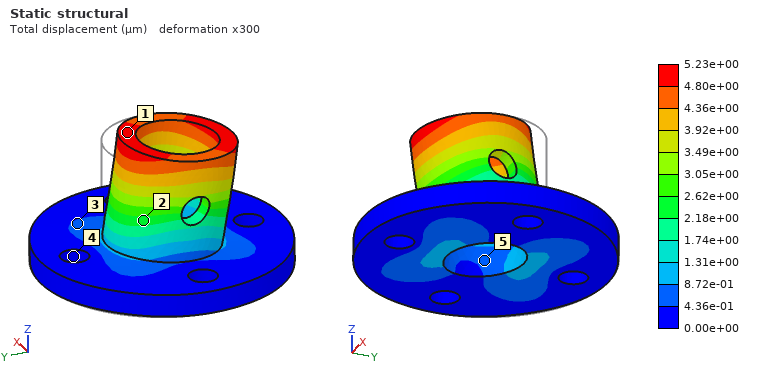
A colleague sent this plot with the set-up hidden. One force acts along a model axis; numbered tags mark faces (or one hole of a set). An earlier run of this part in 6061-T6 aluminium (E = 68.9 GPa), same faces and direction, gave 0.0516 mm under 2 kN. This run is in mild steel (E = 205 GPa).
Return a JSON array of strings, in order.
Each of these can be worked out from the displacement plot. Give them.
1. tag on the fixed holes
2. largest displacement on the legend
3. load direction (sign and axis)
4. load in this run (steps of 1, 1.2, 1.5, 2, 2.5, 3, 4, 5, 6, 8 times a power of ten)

["4", "5.23e+00 µm", "-Y", "600 N"]
